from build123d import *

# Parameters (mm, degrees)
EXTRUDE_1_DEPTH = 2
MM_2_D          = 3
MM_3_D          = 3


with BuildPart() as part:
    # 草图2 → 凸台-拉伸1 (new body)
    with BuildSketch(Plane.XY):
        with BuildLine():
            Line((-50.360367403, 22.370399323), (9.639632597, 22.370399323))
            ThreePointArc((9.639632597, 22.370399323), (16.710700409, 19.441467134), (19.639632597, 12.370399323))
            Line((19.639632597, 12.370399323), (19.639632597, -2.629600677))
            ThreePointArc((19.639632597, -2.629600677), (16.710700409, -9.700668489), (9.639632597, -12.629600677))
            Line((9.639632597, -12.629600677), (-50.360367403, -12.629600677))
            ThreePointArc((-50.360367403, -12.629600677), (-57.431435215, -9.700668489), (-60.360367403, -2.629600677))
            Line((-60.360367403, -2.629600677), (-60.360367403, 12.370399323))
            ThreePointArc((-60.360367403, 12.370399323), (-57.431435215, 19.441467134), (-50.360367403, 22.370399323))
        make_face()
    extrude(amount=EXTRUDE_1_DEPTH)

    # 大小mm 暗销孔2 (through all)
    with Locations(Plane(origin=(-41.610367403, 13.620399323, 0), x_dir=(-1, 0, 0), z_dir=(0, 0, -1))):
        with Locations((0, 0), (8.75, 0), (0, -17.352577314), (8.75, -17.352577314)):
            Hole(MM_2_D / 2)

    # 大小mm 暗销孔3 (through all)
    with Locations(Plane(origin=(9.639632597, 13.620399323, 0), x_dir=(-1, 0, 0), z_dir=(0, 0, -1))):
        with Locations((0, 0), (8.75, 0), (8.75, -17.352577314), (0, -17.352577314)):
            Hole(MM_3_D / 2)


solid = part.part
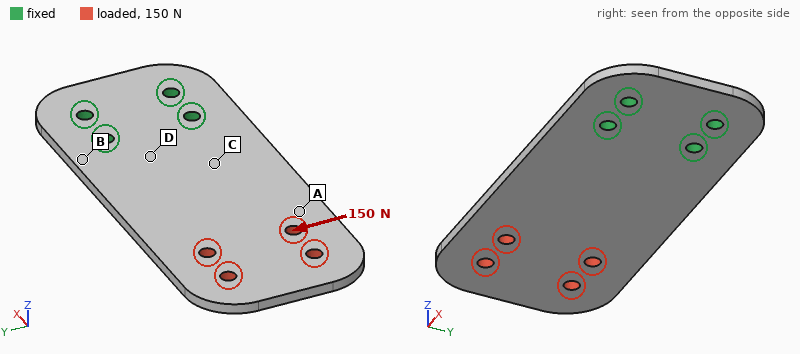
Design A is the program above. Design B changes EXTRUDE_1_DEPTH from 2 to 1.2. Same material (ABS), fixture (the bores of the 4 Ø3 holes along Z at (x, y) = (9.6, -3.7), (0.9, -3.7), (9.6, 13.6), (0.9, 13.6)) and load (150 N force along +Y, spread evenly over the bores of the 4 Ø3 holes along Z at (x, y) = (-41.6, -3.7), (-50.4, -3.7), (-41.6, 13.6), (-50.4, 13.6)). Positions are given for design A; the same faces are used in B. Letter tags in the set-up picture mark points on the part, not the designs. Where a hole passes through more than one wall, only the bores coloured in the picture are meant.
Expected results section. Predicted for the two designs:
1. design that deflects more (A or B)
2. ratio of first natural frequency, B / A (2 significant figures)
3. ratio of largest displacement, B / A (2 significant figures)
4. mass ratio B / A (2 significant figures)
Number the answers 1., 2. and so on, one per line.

1. B
2. 0.61
3. 1.7
4. 0.60
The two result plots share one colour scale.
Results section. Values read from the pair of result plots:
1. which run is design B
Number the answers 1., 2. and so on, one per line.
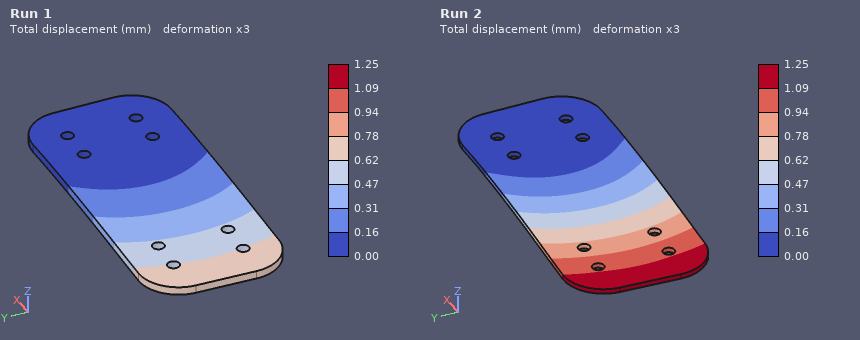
1. Run 2
